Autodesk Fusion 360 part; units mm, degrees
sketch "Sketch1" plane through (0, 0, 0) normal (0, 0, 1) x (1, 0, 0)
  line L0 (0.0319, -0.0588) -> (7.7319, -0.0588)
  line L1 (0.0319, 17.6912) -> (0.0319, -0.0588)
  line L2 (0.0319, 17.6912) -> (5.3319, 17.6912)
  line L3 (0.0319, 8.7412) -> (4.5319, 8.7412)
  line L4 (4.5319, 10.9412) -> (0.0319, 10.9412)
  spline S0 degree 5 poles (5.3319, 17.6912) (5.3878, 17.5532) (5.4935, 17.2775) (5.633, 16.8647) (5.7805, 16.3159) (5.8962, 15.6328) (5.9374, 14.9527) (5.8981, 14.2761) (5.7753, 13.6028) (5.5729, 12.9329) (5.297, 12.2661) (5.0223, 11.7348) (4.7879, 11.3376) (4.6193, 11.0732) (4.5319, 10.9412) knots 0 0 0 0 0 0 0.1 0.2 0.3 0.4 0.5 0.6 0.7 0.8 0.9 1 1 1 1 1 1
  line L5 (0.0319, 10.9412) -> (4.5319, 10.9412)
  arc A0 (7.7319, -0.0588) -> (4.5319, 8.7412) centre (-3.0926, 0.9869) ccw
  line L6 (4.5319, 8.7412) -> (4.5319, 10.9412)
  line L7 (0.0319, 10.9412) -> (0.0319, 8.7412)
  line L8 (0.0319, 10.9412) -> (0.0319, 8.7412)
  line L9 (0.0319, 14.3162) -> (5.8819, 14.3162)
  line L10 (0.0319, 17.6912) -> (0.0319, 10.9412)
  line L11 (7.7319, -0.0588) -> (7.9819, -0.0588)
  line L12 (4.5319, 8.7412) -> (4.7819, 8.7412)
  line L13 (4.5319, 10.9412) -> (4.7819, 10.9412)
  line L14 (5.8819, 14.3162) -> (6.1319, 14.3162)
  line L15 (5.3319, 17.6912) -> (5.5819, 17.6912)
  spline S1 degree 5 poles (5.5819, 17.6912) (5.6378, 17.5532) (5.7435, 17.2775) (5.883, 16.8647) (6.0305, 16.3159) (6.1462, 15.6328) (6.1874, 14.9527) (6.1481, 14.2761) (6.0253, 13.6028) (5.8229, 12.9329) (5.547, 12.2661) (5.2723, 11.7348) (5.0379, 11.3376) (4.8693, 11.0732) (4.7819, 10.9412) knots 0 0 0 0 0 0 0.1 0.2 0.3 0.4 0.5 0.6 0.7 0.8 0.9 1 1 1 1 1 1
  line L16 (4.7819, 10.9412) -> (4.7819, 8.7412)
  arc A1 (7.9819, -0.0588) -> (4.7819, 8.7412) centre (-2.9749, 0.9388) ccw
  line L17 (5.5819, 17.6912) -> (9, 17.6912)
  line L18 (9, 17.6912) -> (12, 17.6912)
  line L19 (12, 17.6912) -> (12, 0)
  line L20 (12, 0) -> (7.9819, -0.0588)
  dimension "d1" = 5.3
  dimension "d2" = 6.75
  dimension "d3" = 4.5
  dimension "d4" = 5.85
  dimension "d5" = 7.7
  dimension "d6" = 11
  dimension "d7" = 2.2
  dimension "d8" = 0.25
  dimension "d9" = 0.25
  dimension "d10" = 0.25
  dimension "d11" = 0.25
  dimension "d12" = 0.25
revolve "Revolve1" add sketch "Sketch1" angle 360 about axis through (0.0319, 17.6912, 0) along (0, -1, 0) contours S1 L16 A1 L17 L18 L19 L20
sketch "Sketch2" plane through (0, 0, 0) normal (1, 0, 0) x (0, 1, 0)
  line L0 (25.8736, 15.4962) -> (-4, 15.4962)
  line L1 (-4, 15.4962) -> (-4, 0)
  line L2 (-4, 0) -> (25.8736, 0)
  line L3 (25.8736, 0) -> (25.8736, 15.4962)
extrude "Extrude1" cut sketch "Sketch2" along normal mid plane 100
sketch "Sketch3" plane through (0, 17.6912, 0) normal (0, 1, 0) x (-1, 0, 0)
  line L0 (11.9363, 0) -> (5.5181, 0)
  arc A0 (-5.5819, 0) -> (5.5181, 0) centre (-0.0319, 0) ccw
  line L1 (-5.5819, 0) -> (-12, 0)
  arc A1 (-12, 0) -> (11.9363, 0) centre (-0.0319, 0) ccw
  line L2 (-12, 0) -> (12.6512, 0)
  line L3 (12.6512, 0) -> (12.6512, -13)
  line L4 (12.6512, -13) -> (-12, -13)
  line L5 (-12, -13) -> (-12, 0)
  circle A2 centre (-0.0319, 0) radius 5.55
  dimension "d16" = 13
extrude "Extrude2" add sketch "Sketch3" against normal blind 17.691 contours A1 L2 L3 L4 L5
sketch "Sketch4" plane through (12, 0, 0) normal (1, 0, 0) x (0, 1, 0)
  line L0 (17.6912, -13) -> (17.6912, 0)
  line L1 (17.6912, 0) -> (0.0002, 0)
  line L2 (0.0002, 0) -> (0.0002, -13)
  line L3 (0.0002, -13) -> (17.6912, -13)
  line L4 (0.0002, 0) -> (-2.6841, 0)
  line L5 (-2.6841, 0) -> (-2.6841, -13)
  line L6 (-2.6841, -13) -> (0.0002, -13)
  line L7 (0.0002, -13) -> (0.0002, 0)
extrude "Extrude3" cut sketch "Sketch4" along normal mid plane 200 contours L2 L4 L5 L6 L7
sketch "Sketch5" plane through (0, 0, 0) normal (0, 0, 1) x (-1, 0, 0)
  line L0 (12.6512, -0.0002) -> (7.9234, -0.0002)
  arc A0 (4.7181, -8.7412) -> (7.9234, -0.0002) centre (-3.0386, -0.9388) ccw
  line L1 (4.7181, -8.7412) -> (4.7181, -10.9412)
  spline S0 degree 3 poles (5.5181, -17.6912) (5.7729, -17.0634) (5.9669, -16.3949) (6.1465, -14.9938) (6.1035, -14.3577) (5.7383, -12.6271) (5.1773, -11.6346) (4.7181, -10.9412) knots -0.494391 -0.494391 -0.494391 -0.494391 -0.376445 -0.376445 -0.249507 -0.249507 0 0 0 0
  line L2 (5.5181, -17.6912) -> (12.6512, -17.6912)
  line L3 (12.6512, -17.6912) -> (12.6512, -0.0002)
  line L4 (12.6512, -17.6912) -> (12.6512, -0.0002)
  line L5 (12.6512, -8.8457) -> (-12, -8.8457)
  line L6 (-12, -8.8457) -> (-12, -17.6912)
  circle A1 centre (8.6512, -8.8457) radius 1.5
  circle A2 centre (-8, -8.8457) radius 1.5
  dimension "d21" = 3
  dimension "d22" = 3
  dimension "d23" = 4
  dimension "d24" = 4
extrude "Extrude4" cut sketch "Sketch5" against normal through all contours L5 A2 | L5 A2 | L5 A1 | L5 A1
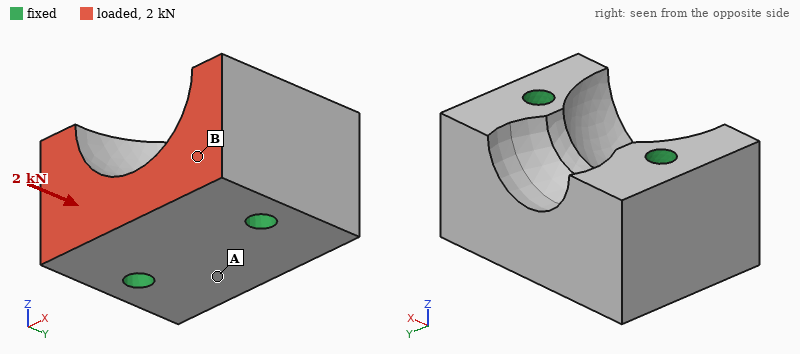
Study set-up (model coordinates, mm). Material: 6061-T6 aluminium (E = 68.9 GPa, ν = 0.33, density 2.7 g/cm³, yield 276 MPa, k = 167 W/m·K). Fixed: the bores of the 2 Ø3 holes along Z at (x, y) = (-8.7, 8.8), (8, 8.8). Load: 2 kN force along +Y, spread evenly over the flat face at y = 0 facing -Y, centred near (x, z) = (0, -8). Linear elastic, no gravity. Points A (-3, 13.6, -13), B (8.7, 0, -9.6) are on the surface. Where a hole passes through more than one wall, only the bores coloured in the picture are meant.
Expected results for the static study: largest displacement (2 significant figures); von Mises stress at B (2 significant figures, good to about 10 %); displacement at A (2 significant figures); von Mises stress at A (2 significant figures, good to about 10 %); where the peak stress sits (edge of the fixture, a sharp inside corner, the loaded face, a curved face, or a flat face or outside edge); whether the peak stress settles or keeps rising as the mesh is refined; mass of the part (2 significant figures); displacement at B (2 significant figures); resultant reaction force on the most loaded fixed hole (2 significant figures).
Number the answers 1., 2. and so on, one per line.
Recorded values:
1. 1.9 µm
2. 9.9 MPa
3. 0.61 µm
4. 3.1 MPa
5. edge of the fixture
6. keeps rising
7. 12 g
8. 1.3 µm
9. 1.0 kN
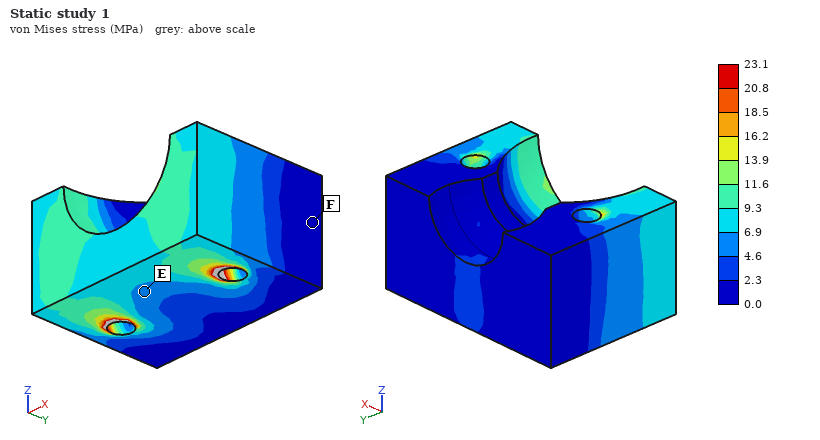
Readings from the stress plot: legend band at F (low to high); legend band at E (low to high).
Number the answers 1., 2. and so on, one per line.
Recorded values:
1. 0.0 to 2.3 MPa
2. 4.6 to 6.9 MPa
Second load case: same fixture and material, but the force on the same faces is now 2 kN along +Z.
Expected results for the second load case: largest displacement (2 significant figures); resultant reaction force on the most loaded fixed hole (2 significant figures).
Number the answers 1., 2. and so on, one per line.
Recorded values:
1. 8.9 µm
2. 1.0 kN
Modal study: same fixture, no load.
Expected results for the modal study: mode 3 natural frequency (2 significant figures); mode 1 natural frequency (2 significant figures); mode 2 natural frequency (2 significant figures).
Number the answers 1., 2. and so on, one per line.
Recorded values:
1. 65 kHz
2. 59 kHz
3. 65 kHz
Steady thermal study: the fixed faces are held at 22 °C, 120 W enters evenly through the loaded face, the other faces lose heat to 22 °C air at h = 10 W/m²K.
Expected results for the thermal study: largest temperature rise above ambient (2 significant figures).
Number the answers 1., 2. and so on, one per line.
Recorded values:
1. 29 K
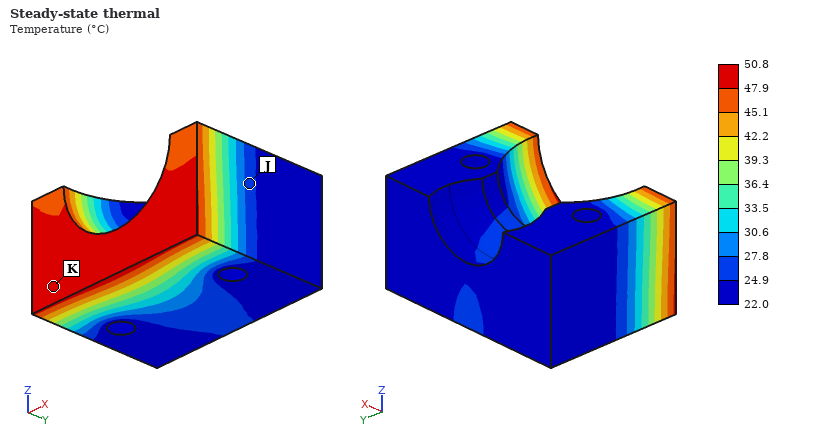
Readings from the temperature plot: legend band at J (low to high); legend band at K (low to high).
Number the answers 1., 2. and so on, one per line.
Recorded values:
1. 24.9 to 27.8 °C
2. 47.9 to 50.8 °C
